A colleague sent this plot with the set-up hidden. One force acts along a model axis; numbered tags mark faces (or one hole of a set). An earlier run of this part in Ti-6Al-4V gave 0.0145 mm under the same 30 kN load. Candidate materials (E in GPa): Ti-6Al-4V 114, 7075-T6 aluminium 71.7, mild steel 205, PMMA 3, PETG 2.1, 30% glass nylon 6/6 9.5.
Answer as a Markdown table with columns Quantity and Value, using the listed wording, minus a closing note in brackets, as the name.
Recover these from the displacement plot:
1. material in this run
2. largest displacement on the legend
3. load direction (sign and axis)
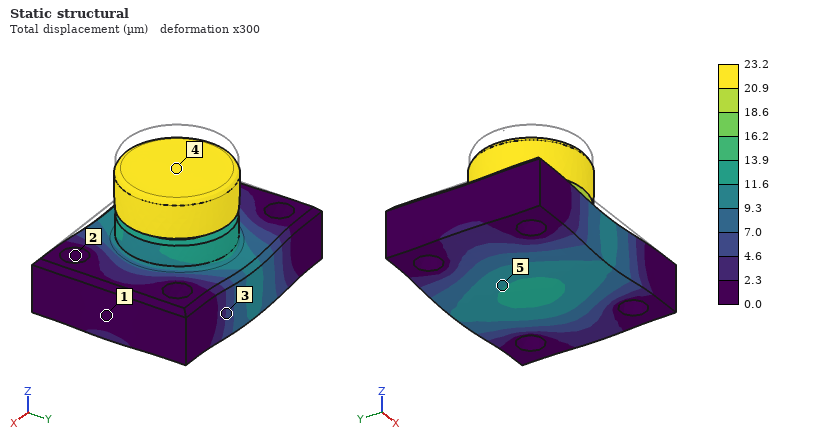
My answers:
| Quantity | Value |
|---|---|
| material in this run | 7075-T6 aluminium |
| largest displacement on the legend | 23.2 µm |
| load direction | -Z |
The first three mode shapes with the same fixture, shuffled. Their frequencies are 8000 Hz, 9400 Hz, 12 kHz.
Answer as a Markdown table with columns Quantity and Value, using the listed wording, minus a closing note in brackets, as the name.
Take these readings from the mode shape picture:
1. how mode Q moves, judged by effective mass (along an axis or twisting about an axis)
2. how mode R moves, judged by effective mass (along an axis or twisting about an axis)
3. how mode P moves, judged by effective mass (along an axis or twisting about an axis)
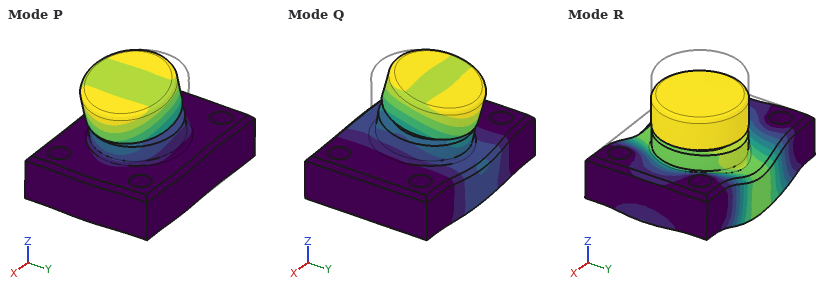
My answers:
| Quantity | Value |
|---|---|
| how mode Q moves, judged by effective mass | along Y |
| how mode R moves, judged by effective mass | along Z |
| how mode P moves, judged by effective mass | along X |
